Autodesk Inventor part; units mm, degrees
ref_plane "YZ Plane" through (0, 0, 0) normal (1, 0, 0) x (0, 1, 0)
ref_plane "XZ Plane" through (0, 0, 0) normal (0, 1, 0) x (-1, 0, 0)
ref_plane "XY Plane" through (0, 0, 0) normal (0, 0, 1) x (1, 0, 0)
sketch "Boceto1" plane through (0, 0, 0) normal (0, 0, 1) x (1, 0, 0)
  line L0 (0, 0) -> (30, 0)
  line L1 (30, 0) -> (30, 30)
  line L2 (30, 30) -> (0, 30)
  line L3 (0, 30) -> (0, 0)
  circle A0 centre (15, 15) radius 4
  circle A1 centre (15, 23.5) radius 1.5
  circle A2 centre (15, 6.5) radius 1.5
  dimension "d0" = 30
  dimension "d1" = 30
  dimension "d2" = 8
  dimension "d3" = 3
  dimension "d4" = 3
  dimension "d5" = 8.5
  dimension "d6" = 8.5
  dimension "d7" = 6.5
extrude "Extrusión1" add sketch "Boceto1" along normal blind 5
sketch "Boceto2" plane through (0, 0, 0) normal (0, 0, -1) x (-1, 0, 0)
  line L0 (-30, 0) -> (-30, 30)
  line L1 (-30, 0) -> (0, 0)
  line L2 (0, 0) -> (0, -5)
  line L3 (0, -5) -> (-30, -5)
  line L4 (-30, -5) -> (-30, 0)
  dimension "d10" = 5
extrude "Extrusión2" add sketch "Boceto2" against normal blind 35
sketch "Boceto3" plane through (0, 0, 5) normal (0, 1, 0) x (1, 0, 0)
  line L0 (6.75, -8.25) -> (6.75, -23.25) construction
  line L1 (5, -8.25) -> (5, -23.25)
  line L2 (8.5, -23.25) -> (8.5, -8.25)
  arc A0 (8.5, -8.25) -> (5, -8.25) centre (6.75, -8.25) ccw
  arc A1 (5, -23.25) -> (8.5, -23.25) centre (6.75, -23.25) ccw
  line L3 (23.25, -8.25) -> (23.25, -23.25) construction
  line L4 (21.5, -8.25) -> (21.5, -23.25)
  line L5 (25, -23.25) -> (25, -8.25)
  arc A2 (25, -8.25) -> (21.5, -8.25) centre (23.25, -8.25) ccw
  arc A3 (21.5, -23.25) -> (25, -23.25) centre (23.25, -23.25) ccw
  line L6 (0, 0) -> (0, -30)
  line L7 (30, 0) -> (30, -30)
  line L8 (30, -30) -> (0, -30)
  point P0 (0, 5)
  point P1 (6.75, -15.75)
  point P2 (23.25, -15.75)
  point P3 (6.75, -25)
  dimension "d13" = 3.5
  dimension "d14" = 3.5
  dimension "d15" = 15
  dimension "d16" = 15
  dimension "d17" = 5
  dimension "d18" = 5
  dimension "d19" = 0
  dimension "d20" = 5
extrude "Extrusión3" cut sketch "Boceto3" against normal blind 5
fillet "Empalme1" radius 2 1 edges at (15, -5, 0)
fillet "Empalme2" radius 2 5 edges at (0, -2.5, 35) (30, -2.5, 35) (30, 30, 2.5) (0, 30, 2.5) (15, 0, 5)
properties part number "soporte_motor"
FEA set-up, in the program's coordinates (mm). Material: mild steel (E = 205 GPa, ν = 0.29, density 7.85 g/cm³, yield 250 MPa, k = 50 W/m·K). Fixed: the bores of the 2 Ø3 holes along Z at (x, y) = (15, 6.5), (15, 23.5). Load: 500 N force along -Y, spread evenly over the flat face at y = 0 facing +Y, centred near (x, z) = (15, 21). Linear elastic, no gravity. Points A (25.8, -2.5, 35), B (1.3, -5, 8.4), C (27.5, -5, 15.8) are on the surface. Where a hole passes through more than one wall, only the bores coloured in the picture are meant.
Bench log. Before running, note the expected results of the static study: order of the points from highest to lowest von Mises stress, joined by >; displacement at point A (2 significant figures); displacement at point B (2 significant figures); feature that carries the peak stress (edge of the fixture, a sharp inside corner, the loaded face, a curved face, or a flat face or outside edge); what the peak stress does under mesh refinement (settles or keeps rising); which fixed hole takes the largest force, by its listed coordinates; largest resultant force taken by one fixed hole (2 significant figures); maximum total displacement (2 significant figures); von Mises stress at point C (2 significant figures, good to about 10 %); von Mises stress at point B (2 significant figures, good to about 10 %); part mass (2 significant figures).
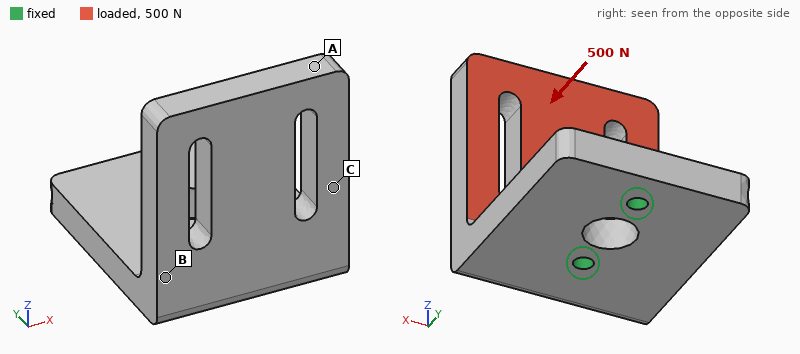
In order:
B > C > A
80 µm
16 µm
edge of the fixture
keeps rising
(15, 6.5)
480 N
81 µm
36 MPa
53 MPa
69 g
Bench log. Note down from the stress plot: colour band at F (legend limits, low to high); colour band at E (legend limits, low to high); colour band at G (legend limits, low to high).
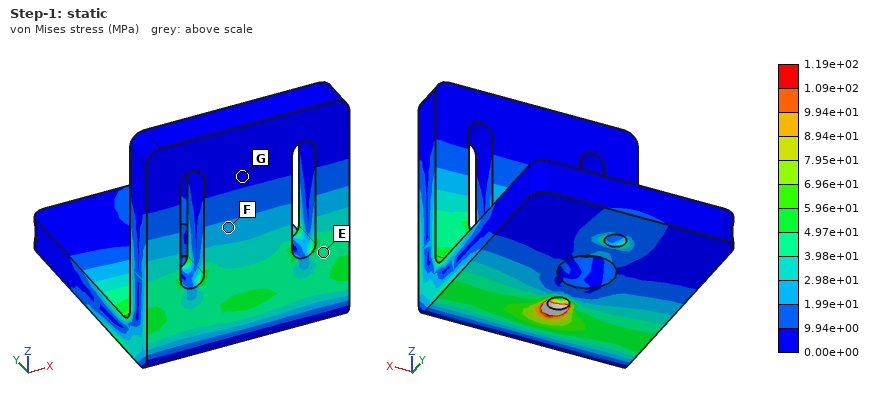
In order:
1.99e+01 to 2.98e+01 MPa
3.98e+01 to 4.97e+01 MPa
0.00e+00 to 9.94e+00 MPa
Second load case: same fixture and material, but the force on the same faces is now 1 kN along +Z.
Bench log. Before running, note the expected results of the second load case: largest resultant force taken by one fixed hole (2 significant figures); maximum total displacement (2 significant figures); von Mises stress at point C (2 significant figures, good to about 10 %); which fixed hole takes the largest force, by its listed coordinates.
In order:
1.1 kN
8.3 µm
12 MPa
(15, 6.5)
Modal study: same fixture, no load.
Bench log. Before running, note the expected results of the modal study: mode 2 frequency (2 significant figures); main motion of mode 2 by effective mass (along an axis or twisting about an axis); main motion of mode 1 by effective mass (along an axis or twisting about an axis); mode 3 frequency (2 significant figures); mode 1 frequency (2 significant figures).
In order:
3700 Hz
along X
along Y
8100 Hz
2800 Hz
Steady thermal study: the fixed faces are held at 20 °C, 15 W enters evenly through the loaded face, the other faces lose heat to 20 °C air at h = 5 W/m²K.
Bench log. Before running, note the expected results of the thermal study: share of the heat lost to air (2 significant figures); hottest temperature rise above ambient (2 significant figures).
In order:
3.5 %
63 K
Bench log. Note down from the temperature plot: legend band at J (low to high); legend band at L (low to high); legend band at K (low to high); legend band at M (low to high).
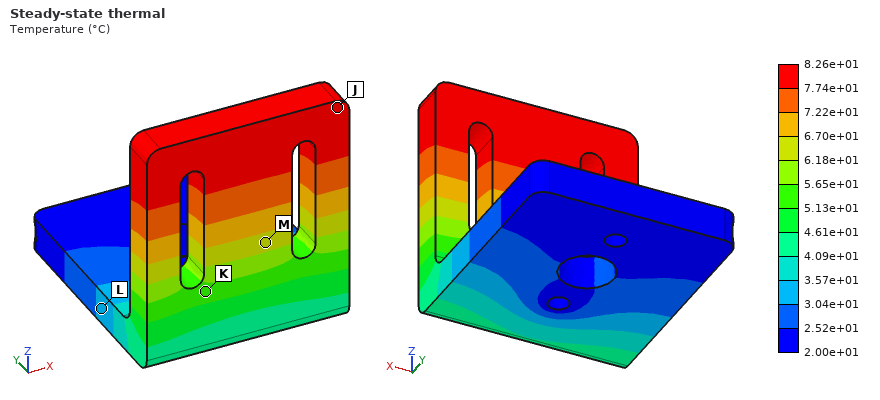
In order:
7.74e+01 to 8.26e+01 °C
3.04e+01 to 3.57e+01 °C
5.13e+01 to 5.65e+01 °C
6.18e+01 to 6.70e+01 °C
